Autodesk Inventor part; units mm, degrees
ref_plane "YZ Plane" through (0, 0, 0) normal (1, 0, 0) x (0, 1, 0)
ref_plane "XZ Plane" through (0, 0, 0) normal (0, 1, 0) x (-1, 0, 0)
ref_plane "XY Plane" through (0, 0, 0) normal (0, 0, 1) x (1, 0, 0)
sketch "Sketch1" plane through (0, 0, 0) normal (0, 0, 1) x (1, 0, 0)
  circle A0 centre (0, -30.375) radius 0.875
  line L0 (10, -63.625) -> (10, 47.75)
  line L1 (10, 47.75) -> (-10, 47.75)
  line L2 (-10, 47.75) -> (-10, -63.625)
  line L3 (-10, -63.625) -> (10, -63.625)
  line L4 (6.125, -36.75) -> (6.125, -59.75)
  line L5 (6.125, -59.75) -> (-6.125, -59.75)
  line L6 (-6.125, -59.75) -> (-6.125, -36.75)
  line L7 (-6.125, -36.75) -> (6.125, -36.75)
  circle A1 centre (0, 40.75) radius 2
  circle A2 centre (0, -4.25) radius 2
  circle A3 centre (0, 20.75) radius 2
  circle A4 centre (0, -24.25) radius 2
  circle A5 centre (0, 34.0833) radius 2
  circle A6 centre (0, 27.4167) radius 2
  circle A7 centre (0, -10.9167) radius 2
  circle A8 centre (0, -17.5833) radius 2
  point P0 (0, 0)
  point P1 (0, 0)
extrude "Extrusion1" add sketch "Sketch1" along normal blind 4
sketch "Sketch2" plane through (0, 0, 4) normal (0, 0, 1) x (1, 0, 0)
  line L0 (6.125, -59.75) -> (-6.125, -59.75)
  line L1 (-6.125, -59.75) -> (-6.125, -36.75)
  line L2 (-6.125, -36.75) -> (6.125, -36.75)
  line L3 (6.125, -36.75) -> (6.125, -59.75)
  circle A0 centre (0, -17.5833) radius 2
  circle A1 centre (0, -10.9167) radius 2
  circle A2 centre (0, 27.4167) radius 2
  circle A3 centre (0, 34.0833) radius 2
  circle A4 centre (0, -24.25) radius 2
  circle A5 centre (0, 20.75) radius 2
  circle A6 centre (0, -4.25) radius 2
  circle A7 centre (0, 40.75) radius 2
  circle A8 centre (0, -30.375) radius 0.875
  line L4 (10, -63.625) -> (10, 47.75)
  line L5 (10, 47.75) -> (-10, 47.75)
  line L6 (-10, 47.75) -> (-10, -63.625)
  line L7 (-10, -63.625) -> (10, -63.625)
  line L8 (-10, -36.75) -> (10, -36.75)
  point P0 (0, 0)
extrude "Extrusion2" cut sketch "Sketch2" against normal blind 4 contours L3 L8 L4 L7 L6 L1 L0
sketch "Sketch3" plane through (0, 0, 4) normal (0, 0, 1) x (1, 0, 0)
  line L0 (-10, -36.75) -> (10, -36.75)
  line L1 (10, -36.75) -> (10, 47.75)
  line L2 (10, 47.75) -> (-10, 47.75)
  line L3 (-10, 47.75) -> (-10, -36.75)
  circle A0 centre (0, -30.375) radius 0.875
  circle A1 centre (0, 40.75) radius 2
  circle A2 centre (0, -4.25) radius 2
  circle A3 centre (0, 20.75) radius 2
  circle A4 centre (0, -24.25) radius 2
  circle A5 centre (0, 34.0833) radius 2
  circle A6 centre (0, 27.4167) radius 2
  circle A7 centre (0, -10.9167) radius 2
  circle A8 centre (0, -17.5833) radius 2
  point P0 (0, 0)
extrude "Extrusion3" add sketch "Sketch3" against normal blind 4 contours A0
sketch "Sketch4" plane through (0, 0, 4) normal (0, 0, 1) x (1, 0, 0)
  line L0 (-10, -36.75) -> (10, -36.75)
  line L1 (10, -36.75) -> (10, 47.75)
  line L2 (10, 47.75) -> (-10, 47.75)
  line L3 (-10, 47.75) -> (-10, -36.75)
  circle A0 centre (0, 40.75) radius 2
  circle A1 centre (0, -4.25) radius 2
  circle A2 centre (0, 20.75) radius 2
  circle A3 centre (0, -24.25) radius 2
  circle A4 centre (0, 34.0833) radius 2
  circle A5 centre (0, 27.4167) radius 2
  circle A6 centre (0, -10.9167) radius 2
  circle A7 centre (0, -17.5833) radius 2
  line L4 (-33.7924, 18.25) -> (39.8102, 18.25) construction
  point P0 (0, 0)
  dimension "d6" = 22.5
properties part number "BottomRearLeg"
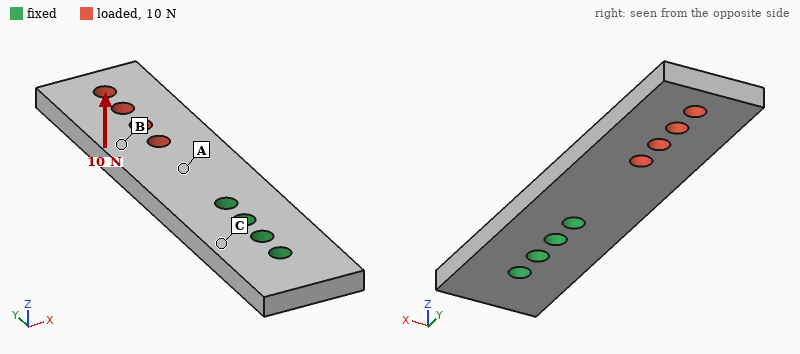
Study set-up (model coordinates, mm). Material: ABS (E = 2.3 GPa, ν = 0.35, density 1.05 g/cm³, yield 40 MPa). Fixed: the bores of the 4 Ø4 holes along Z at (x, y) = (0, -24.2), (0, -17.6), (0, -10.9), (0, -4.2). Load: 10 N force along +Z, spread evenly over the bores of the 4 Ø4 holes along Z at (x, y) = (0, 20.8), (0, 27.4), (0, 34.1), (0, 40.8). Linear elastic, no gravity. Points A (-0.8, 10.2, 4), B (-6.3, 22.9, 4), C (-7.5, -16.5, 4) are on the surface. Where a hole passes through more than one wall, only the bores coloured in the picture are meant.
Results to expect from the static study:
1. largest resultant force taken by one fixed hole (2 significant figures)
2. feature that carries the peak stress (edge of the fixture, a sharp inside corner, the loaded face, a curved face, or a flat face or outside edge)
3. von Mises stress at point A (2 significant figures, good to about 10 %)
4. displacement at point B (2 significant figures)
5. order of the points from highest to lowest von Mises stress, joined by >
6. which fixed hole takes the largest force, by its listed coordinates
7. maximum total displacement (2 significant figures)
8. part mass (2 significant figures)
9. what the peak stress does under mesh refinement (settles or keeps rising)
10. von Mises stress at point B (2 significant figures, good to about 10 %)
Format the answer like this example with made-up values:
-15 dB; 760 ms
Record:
25 N; edge of the fixture; 3.6 MPa; 0.38 mm; A > B > C; (0, -4.2); 1.0 mm; 6.7 g; keeps rising; 1.9 MPa
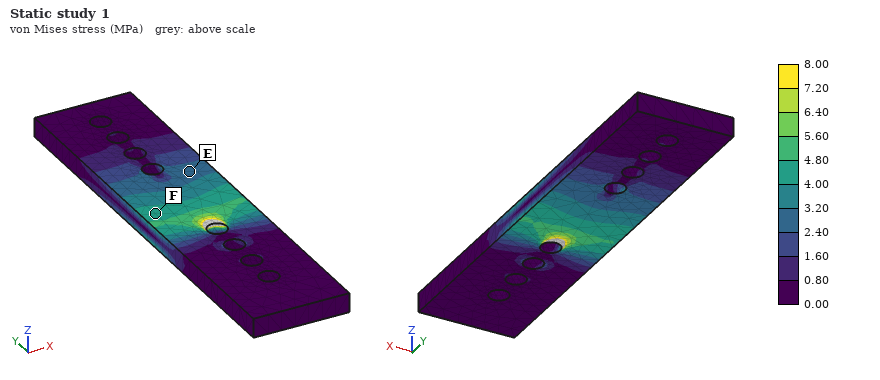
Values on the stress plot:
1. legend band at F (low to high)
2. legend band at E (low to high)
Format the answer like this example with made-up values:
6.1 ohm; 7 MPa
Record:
4.00 to 4.80 MPa; 2.40 to 3.20 MPa
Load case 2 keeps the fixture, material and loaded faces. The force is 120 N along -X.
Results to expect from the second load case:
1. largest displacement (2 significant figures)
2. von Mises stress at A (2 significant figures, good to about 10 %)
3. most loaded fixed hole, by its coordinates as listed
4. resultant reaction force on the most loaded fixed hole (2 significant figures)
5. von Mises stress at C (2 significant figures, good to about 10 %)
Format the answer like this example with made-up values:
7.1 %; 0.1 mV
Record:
0.89 mm; 4.1 MPa; (0, -4.2); 330 N; 3.1 MPa
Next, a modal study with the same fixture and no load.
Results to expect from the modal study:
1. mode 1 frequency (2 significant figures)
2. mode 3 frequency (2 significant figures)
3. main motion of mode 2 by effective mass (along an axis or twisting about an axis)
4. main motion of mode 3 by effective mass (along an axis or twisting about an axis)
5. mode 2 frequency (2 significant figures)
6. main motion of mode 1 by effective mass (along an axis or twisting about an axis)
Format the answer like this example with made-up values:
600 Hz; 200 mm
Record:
370 Hz; 1600 Hz; along X; twisting about Y; 1300 Hz; along Z
